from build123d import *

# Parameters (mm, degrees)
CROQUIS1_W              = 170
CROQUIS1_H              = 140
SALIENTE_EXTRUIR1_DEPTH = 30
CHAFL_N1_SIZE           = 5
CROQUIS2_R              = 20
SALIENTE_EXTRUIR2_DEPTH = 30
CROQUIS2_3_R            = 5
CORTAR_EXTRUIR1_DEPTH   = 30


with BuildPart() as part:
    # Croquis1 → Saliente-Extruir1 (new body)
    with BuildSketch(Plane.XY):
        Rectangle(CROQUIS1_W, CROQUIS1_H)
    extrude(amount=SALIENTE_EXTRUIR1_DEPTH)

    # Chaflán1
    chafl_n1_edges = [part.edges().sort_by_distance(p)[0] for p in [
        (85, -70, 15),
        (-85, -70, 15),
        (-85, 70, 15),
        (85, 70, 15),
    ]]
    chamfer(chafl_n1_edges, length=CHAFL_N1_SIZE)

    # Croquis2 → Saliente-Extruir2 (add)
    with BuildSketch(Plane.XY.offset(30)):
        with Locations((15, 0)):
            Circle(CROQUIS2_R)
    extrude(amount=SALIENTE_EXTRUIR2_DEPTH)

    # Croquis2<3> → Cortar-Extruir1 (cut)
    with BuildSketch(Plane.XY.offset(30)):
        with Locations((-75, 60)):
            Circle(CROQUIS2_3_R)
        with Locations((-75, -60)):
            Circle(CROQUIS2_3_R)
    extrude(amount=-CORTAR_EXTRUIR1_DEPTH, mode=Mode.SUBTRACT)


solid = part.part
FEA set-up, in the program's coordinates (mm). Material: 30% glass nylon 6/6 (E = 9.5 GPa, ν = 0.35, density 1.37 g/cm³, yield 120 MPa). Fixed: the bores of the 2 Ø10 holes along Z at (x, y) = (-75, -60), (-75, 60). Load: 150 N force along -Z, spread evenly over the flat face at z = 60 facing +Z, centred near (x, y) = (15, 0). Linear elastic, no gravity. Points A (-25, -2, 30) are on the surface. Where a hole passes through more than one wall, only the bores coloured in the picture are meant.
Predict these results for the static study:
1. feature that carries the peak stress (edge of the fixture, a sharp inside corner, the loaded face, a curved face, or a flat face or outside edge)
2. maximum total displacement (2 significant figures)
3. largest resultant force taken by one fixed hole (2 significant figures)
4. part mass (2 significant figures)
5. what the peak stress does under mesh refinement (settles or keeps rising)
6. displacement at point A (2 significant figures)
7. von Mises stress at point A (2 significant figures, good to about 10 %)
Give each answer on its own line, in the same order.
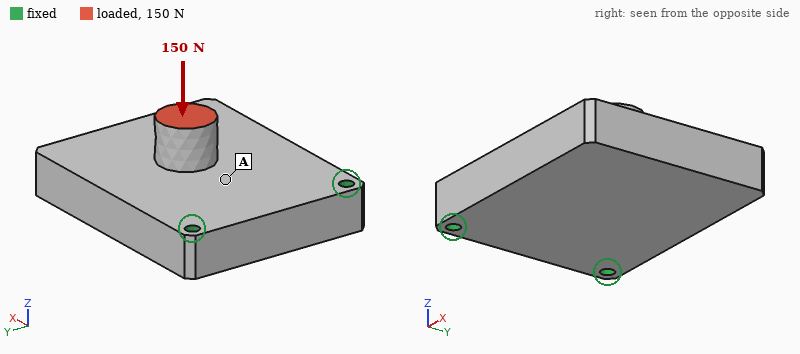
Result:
edge of the fixture
49 µm
75 N
1.0 kg
keeps rising
13 µm
0.27 MPa
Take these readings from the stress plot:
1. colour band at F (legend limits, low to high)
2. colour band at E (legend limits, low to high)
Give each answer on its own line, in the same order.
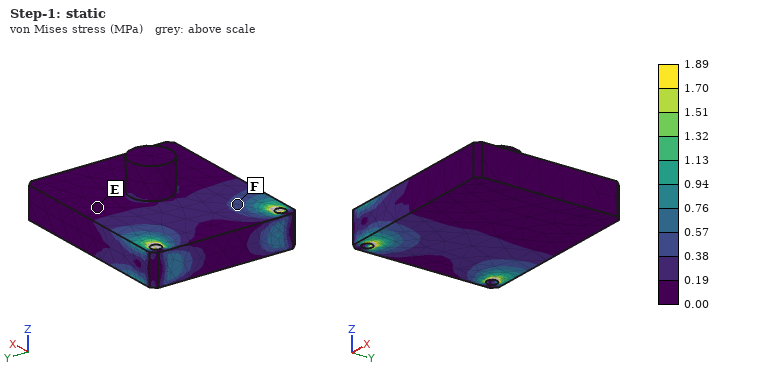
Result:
0.38 to 0.57 MPa
0.00 to 0.19 MPa
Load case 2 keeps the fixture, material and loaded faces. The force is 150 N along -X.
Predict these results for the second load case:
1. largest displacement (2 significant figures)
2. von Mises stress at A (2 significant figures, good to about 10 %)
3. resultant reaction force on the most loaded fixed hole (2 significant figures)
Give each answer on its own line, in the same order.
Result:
34 µm
0.33 MPa
80 N
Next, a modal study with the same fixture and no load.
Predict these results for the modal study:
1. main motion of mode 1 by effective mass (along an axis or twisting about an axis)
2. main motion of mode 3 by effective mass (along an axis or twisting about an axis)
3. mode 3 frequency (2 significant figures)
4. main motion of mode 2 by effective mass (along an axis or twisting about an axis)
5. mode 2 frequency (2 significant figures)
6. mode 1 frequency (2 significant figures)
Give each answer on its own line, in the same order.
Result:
along Z
along Y
1500 Hz
twisting about X
1200 Hz
370 Hz
